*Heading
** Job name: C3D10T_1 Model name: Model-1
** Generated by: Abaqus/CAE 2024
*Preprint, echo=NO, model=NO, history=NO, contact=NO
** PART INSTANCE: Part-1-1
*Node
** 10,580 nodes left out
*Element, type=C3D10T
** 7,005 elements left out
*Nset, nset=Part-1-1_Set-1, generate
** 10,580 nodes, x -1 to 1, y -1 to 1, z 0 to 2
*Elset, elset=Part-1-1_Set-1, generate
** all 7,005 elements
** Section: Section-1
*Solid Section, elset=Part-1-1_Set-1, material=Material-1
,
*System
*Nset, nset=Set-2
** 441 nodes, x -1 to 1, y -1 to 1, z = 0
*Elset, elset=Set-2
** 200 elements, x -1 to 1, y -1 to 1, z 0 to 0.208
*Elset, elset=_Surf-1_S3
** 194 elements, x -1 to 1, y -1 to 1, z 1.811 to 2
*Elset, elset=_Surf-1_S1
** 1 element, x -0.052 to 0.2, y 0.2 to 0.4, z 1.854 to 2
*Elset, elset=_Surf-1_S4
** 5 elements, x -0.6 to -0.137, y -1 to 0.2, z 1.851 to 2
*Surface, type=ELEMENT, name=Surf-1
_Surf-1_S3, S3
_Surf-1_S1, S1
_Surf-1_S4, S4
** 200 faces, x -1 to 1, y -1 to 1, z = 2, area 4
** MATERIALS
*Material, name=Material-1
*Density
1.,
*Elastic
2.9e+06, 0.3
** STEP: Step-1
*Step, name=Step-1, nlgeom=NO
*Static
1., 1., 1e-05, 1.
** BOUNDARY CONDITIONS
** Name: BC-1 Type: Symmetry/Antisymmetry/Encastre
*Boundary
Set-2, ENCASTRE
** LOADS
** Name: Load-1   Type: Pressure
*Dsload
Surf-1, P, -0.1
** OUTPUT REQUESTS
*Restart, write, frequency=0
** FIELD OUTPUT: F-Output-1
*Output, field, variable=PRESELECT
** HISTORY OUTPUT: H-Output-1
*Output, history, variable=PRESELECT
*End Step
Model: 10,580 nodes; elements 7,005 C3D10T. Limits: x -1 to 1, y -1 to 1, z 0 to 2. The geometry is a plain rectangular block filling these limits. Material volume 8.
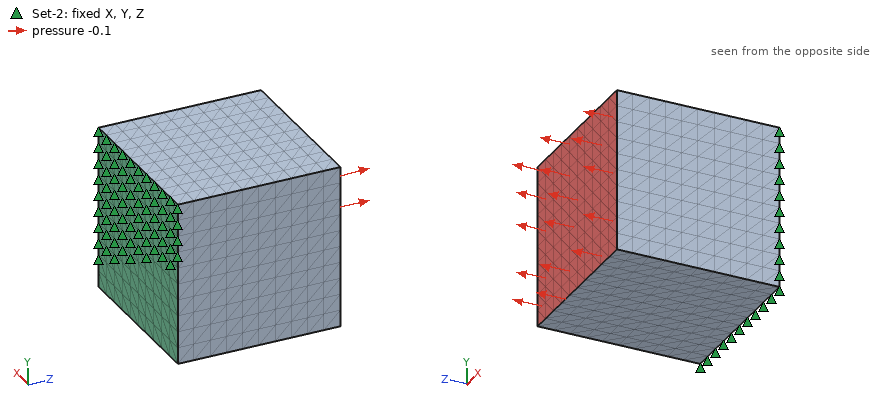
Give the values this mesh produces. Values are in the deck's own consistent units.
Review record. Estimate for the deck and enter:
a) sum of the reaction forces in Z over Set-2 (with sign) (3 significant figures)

-0.400
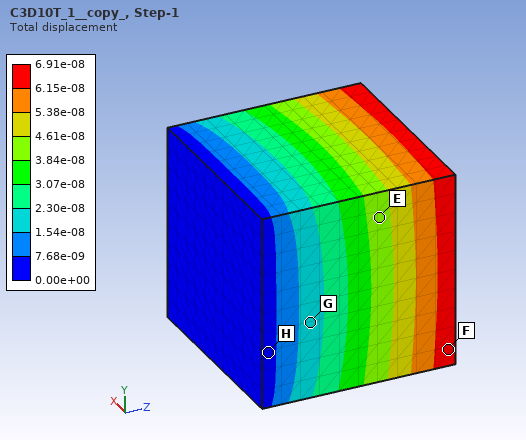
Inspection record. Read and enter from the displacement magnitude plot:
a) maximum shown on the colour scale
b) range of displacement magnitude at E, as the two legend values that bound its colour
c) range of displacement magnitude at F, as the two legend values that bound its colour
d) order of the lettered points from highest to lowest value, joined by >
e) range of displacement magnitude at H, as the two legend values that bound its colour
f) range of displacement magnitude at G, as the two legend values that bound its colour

6.91e-08
3.84e-08 to 4.61e-08
6.15e-08 to 6.91e-08
F > E > G > H
0.00e+00 to 7.68e-09
1.54e-08 to 2.30e-08
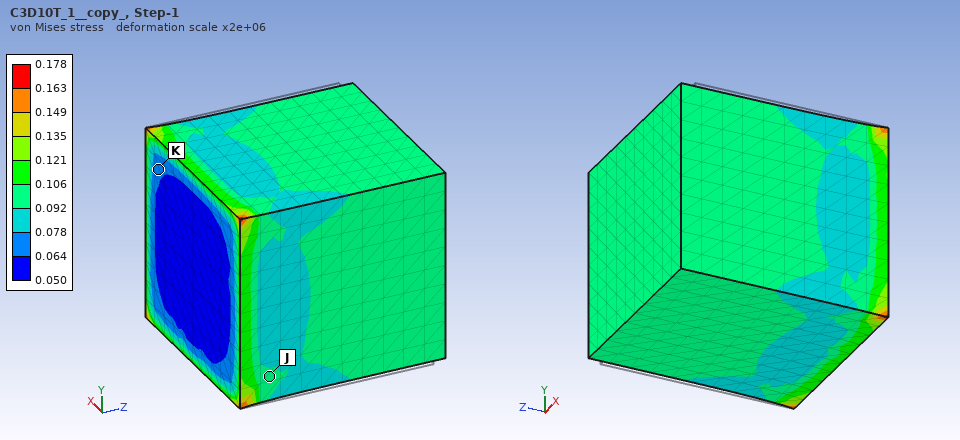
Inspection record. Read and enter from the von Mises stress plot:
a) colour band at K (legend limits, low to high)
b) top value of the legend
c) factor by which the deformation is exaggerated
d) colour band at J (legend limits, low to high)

0.064 to 0.078
0.178
2e+06
0.092 to 0.106
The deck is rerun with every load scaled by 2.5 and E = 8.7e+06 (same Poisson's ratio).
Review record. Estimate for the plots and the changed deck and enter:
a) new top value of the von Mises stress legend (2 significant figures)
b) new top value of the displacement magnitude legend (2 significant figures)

0.44
5.8e-08
